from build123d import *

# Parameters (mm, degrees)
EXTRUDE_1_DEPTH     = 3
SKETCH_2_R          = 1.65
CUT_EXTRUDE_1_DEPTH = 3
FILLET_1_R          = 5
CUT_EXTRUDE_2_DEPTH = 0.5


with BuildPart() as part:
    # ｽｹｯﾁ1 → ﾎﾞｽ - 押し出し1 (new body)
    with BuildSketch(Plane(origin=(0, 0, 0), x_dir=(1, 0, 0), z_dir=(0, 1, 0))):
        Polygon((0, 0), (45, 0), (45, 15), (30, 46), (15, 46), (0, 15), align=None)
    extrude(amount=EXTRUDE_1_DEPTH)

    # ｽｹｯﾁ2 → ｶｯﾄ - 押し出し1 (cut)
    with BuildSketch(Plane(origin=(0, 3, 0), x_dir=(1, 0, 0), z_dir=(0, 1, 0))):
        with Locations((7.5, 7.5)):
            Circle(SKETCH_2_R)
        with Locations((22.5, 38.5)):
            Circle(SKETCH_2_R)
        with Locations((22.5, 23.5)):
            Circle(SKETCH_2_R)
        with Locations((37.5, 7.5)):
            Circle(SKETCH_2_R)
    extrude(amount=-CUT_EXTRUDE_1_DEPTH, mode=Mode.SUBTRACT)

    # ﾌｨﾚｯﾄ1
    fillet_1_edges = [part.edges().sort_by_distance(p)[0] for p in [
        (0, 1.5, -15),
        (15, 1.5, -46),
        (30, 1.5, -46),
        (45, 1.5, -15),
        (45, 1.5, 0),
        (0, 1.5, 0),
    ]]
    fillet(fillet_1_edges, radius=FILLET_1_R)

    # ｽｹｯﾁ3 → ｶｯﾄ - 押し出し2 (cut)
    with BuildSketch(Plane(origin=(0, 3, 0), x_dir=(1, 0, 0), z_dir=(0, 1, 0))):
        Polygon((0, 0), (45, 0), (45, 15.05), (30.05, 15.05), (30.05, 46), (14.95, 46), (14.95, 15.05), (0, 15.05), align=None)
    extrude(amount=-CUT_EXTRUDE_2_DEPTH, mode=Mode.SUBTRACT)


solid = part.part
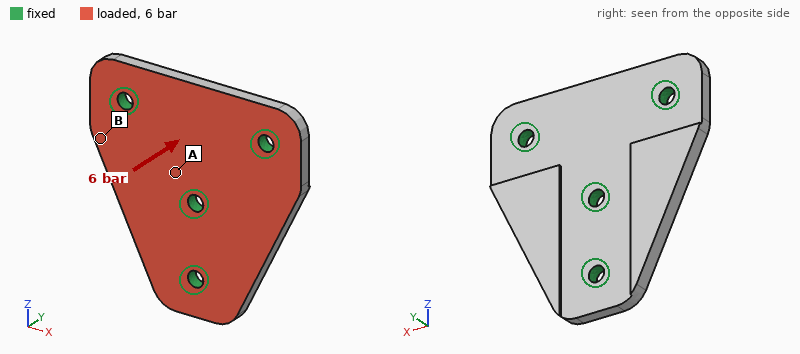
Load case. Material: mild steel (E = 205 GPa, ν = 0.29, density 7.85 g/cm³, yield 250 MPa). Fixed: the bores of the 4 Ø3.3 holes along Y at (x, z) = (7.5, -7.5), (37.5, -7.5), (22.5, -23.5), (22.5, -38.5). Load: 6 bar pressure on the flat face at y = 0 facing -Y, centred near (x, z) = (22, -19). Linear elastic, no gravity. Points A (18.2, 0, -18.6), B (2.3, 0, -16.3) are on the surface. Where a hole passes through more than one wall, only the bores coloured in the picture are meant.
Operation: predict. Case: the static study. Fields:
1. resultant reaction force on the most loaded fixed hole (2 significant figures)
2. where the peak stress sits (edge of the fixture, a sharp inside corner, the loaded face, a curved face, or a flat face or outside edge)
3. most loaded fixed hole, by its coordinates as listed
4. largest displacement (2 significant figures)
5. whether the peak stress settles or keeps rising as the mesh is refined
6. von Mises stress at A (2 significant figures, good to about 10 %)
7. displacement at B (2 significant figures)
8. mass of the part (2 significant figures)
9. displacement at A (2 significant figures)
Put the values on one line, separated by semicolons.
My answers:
260 N; edge of the fixture; (22.5, -23.5); 7.0 µm; keeps rising; 17 MPa; 4.0 µm; 32 g; 1.2 µm
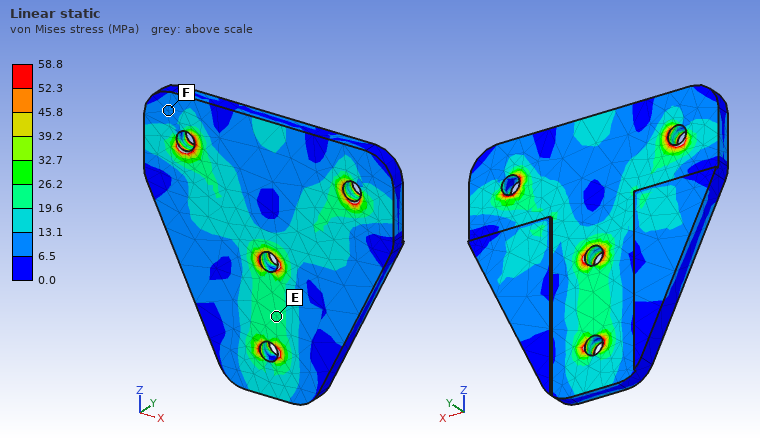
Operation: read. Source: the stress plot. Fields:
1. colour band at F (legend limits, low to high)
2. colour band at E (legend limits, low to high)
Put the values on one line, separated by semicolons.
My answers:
6.5 to 13.1 MPa; 19.6 to 26.2 MPa
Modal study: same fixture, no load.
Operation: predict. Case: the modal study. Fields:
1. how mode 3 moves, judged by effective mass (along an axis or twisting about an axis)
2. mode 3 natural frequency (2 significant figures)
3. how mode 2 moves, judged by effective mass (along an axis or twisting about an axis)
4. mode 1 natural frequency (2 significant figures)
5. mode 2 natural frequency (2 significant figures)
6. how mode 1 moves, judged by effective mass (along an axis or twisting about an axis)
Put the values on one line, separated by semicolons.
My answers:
along Y; 16 kHz; along Y; 12 kHz; 12 kHz; twisting about Z
